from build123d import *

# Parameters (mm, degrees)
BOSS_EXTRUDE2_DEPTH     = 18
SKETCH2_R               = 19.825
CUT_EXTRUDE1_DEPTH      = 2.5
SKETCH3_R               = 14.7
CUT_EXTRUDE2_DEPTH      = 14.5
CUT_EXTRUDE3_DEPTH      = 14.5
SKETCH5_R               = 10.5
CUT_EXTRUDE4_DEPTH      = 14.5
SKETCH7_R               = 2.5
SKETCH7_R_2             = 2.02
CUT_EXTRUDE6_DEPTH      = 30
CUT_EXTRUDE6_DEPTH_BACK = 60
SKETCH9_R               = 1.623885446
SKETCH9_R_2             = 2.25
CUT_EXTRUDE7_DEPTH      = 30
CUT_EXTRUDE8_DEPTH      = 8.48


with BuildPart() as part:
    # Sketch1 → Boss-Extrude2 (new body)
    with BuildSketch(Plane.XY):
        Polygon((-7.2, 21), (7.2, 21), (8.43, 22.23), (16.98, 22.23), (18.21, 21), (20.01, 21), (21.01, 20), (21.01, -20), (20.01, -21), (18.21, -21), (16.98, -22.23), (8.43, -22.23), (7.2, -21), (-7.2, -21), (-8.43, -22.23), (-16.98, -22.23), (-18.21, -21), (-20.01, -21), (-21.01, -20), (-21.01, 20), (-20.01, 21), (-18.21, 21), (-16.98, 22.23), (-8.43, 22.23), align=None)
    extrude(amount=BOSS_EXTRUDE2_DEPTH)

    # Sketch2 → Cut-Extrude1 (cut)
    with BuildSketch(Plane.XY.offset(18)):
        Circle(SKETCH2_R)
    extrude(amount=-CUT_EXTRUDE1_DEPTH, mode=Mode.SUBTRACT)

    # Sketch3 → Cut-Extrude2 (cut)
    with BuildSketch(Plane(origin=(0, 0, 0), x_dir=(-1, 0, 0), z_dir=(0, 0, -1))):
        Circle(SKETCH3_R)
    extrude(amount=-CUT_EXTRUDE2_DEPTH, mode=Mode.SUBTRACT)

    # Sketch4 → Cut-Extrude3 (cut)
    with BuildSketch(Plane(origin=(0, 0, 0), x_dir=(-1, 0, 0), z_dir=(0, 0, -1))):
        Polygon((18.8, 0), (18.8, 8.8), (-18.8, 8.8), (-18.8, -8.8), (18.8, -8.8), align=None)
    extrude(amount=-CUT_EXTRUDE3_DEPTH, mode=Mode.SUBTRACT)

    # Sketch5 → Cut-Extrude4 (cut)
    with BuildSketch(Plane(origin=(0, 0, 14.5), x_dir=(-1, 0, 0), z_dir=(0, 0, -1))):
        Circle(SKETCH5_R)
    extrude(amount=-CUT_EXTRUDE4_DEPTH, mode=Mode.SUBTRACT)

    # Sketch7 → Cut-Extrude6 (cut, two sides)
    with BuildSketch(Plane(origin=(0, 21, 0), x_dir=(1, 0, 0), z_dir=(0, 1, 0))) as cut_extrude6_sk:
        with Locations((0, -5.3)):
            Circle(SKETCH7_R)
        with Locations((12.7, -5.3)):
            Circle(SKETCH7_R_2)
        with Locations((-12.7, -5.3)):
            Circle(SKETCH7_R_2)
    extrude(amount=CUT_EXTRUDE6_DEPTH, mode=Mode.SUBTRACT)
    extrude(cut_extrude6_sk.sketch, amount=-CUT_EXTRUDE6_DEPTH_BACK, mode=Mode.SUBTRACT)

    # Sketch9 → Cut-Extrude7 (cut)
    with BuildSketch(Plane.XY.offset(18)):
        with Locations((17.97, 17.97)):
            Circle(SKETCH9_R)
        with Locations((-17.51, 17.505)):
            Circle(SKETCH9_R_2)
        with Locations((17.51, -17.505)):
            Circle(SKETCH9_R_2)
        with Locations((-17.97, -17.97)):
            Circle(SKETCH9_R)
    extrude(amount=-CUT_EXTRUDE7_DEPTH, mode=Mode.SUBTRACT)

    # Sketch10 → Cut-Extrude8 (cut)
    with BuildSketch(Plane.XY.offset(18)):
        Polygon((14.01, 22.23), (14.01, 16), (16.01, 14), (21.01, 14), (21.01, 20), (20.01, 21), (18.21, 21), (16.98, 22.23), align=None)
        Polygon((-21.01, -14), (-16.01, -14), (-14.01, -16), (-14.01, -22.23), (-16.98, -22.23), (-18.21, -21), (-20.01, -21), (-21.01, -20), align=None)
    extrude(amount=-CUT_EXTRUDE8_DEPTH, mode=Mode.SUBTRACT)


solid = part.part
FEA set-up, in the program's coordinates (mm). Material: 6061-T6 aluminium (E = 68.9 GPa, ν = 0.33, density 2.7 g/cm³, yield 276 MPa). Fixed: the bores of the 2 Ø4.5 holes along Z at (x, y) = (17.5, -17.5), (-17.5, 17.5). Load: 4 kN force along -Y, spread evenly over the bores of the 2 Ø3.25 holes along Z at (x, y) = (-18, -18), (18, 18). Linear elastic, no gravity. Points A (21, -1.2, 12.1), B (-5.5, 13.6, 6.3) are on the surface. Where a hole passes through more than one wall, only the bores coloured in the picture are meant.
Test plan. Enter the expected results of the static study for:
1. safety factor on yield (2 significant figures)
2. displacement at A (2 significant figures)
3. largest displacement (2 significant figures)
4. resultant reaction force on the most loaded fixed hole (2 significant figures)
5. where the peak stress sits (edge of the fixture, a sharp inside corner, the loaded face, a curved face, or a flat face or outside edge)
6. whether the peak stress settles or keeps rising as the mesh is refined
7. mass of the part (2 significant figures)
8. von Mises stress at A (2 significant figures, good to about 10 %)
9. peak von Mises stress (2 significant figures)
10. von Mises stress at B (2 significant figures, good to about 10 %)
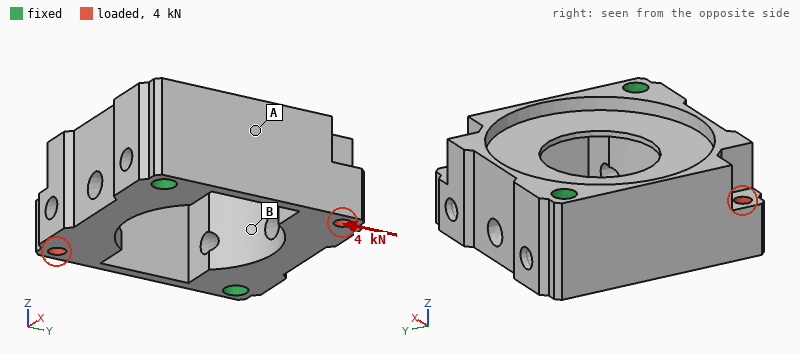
2.8
5.8 µm
37 µm
2.0 kN
a flat face or outside edge
settles
38 g
29 MPa
99 MPa
14 MPa
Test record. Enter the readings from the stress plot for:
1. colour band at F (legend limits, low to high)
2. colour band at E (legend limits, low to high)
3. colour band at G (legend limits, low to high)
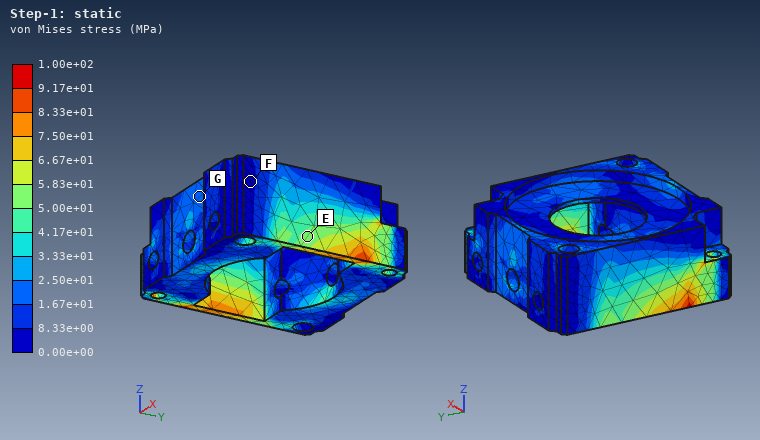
0.00e+00 to 8.33e+00 MPa
5.00e+01 to 5.83e+01 MPa
1.67e+01 to 2.50e+01 MPa
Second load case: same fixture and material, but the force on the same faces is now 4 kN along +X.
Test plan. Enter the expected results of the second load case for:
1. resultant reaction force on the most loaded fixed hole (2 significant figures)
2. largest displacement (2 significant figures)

2.0 kN
27 µm
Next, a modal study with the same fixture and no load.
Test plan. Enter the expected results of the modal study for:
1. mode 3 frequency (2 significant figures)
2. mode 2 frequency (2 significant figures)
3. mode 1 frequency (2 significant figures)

17 kHz
11 kHz
11 kHz
